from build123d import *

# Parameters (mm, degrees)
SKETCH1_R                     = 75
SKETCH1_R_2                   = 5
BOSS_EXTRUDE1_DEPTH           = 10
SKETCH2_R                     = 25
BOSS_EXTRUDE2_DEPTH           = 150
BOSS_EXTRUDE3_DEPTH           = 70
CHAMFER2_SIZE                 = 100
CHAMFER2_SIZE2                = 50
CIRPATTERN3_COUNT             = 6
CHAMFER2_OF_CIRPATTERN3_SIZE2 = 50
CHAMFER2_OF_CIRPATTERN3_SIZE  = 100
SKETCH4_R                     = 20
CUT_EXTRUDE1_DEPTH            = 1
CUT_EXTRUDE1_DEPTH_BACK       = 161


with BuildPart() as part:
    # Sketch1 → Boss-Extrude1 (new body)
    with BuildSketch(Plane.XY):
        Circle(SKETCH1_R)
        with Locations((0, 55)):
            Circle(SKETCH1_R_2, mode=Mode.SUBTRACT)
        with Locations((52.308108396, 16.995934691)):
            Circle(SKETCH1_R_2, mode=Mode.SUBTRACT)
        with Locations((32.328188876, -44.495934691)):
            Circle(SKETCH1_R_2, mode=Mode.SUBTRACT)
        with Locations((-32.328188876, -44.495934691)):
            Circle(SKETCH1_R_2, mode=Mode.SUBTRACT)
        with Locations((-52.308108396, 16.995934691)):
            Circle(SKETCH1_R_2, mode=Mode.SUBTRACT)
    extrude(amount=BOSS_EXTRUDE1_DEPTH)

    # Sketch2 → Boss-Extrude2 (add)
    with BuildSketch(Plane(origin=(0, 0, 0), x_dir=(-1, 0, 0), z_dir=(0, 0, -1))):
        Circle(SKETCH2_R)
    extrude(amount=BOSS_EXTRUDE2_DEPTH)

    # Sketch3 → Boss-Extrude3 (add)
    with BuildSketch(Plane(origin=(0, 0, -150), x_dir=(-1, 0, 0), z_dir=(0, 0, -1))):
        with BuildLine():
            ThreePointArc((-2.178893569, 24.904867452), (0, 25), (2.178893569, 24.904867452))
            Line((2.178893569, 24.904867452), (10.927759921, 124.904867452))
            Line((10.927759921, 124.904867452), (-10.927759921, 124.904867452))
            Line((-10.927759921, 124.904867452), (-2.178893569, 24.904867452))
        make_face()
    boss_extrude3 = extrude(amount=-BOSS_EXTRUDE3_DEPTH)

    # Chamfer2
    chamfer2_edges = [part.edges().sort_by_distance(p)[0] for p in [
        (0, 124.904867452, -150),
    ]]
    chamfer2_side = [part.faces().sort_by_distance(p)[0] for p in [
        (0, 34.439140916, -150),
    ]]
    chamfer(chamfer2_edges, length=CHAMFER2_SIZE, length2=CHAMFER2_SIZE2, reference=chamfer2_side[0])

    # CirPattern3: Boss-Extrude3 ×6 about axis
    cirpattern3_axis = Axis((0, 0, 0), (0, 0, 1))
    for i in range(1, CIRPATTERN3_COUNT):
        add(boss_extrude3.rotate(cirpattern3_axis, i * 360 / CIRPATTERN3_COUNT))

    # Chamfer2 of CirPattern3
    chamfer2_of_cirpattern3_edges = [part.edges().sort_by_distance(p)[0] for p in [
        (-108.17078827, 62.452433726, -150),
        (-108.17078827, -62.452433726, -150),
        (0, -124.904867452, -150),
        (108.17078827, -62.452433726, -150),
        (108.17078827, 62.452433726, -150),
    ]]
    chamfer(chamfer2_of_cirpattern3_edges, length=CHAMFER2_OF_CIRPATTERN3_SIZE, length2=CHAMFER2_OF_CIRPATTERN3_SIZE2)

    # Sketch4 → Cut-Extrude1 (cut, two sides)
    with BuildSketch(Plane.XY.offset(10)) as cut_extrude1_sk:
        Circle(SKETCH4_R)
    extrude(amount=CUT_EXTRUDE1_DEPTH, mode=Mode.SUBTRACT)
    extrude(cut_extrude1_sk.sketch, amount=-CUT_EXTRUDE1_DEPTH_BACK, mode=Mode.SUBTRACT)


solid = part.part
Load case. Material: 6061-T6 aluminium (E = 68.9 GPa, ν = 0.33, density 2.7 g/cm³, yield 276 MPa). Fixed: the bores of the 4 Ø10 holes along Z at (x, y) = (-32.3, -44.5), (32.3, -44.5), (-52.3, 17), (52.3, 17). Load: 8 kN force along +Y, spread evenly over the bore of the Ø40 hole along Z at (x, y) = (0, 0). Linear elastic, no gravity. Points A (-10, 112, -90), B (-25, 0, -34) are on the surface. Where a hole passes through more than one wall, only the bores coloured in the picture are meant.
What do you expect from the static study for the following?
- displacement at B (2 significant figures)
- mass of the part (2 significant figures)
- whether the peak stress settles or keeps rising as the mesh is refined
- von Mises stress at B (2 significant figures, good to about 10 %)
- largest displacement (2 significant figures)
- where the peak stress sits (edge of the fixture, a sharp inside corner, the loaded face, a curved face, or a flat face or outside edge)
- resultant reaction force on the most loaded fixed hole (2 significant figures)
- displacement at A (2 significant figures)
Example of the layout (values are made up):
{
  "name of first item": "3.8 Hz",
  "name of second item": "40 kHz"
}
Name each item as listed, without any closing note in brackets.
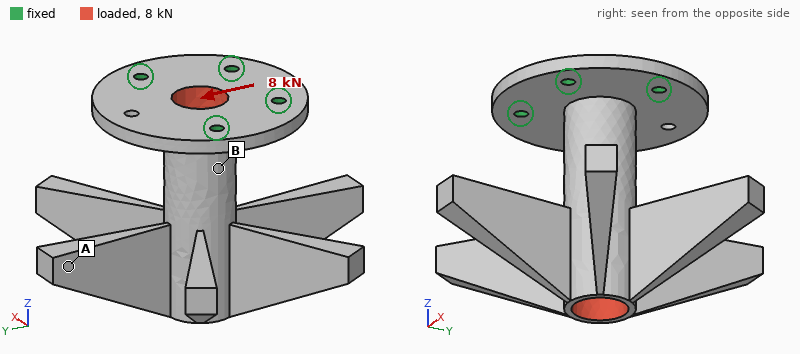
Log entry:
{
  "displacement at B": "0.25 mm",
  "mass of the part": "1.6 kg",
  "whether the peak stress settles or keeps rising as the mesh is refined": "keeps rising",
  "von Mises stress at B": "27 MPa",
  "largest displacement": "1.2 mm",
  "where the peak stress sits": "edge of the fixture",
  "resultant reaction force on the most loaded fixed hole": "5.8 kN",
  "displacement at A": "1.1 mm"
}
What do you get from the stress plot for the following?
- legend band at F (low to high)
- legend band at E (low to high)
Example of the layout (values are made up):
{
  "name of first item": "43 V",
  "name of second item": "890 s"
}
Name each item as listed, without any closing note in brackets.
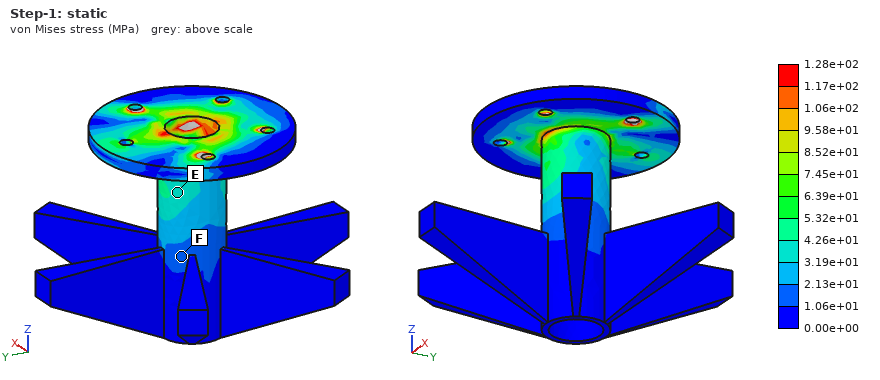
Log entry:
{
  "legend band at F": "1.06e+01 to 2.13e+01 MPa",
  "legend band at E": "3.19e+01 to 4.26e+01 MPa"
}
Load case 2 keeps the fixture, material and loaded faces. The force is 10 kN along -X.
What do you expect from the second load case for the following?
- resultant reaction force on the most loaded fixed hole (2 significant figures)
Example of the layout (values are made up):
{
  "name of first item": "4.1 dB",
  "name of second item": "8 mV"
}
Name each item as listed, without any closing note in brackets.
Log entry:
{
  "resultant reaction force on the most loaded fixed hole": "7.7 kN"
}
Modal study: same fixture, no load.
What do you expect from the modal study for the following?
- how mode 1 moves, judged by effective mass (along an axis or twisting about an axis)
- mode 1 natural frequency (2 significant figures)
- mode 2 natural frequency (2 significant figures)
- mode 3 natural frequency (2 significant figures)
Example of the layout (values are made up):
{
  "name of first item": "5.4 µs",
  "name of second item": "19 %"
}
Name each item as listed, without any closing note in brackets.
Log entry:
{
  "how mode 1 moves, judged by effective mass": "along Y",
  "mode 1 natural frequency": "320 Hz",
  "mode 2 natural frequency": "340 Hz",
  "mode 3 natural frequency": "350 Hz"
}
